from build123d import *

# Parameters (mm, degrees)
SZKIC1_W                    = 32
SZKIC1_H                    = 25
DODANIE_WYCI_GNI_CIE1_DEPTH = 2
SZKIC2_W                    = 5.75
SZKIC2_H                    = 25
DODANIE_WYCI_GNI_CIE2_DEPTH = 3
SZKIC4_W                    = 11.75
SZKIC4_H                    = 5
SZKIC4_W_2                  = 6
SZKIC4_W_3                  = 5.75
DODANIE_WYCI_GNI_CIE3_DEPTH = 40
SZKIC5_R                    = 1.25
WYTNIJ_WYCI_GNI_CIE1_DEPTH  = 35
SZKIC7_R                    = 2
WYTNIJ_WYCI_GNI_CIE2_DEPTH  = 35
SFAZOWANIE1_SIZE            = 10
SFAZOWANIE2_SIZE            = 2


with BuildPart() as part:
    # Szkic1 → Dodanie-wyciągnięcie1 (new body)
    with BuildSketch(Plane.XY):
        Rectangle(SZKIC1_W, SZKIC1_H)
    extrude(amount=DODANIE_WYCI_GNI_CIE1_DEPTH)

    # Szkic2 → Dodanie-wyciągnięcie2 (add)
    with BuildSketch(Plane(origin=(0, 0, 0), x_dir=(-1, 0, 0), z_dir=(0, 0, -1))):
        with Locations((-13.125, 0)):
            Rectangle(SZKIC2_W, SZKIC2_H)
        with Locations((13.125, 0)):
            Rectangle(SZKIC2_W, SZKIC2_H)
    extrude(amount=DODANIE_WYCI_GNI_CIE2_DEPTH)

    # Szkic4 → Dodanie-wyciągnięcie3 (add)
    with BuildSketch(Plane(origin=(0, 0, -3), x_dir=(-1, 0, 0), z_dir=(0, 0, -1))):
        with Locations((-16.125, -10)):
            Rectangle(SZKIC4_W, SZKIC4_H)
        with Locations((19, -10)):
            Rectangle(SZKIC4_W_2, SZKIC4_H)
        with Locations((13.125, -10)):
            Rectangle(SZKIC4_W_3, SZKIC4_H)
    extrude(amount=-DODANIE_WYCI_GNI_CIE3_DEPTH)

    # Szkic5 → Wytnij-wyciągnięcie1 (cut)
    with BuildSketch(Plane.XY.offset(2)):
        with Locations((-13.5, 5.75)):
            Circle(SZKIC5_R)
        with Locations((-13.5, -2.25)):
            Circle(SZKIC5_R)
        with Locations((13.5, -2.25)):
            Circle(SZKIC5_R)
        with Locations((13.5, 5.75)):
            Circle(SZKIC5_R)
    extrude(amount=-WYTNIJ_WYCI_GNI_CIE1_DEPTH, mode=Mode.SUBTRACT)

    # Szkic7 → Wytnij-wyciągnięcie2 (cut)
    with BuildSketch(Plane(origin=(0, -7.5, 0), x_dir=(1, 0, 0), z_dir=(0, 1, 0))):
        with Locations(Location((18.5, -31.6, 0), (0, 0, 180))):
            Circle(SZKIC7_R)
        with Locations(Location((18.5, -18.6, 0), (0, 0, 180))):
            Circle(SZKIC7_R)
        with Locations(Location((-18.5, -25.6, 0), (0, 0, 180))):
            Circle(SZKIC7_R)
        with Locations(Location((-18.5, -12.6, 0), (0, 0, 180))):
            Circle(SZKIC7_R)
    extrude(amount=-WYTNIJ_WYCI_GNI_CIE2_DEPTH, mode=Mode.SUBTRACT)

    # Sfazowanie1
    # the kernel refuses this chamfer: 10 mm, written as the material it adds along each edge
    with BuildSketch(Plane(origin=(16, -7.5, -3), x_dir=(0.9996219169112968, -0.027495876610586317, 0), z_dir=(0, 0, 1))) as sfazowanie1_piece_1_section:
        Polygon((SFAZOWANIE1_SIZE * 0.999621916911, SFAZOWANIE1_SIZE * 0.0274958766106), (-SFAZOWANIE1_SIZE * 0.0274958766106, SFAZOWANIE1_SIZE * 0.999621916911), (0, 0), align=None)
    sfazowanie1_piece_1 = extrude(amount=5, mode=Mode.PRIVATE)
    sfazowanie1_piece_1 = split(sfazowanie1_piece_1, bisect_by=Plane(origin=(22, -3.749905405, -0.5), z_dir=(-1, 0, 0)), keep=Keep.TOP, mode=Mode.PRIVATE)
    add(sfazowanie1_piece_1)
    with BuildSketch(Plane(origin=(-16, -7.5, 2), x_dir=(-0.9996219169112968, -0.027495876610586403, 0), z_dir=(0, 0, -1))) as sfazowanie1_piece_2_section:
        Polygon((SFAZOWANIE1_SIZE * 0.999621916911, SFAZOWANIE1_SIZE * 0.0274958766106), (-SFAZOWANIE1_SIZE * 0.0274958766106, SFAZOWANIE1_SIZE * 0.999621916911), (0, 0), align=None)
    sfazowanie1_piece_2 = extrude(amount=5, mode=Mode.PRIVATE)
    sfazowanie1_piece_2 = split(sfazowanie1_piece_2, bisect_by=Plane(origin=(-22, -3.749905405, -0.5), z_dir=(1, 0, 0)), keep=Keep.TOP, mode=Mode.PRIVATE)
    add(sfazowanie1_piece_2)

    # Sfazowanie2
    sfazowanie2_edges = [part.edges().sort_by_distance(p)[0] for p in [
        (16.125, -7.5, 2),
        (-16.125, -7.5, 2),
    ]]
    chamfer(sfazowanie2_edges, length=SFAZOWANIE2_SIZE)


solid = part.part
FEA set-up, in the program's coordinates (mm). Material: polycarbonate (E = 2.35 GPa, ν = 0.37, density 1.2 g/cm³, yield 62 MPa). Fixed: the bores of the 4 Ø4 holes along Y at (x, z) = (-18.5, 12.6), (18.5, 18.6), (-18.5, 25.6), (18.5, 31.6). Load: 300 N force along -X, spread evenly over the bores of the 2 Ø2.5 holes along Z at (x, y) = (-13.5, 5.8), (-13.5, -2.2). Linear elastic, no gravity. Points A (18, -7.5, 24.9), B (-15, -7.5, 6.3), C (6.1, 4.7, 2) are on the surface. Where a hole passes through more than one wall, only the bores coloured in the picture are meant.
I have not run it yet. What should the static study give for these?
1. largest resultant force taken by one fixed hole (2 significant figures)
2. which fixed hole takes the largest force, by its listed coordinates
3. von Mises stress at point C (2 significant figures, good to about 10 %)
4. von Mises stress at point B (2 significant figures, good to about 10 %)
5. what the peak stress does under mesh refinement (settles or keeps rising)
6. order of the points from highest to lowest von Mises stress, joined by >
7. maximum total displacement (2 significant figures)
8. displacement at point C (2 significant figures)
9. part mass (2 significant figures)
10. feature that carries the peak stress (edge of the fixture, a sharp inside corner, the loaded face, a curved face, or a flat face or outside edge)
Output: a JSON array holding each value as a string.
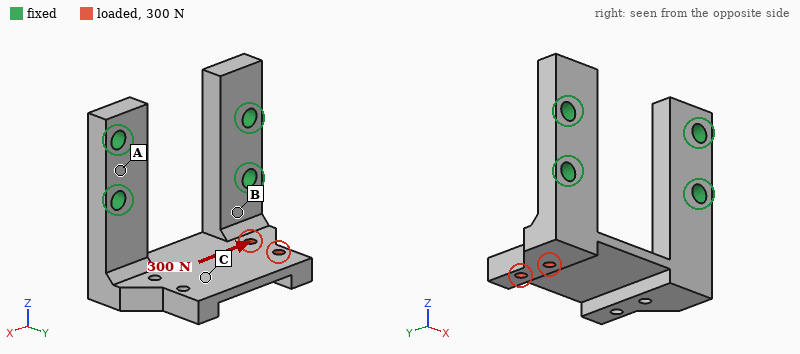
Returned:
["310 N", "(-18.5, 12.6)", "9.0 MPa", "17 MPa", "keeps rising", "B > C > A", "0.77 mm", "0.51 mm", "8.4 g", "edge of the fixture"]
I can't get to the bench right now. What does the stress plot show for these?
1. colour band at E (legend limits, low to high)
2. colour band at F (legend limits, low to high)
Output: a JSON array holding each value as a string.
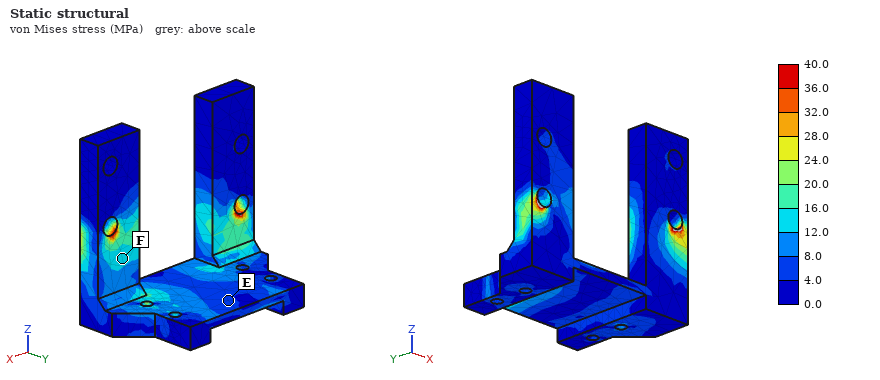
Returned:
["4.0 to 8.0 MPa", "12.0 to 16.0 MPa"]
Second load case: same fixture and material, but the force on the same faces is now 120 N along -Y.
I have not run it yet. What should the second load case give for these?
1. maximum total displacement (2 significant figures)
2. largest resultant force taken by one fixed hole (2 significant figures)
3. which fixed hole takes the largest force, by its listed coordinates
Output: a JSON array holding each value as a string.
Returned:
["0.68 mm", "120 N", "(-18.5, 12.6)"]
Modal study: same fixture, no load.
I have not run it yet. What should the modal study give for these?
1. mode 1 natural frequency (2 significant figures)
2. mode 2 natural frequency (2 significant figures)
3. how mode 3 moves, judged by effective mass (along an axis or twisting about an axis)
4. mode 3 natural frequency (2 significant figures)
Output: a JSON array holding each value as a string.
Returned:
["1100 Hz", "1800 Hz", "along Y", "2600 Hz"]
